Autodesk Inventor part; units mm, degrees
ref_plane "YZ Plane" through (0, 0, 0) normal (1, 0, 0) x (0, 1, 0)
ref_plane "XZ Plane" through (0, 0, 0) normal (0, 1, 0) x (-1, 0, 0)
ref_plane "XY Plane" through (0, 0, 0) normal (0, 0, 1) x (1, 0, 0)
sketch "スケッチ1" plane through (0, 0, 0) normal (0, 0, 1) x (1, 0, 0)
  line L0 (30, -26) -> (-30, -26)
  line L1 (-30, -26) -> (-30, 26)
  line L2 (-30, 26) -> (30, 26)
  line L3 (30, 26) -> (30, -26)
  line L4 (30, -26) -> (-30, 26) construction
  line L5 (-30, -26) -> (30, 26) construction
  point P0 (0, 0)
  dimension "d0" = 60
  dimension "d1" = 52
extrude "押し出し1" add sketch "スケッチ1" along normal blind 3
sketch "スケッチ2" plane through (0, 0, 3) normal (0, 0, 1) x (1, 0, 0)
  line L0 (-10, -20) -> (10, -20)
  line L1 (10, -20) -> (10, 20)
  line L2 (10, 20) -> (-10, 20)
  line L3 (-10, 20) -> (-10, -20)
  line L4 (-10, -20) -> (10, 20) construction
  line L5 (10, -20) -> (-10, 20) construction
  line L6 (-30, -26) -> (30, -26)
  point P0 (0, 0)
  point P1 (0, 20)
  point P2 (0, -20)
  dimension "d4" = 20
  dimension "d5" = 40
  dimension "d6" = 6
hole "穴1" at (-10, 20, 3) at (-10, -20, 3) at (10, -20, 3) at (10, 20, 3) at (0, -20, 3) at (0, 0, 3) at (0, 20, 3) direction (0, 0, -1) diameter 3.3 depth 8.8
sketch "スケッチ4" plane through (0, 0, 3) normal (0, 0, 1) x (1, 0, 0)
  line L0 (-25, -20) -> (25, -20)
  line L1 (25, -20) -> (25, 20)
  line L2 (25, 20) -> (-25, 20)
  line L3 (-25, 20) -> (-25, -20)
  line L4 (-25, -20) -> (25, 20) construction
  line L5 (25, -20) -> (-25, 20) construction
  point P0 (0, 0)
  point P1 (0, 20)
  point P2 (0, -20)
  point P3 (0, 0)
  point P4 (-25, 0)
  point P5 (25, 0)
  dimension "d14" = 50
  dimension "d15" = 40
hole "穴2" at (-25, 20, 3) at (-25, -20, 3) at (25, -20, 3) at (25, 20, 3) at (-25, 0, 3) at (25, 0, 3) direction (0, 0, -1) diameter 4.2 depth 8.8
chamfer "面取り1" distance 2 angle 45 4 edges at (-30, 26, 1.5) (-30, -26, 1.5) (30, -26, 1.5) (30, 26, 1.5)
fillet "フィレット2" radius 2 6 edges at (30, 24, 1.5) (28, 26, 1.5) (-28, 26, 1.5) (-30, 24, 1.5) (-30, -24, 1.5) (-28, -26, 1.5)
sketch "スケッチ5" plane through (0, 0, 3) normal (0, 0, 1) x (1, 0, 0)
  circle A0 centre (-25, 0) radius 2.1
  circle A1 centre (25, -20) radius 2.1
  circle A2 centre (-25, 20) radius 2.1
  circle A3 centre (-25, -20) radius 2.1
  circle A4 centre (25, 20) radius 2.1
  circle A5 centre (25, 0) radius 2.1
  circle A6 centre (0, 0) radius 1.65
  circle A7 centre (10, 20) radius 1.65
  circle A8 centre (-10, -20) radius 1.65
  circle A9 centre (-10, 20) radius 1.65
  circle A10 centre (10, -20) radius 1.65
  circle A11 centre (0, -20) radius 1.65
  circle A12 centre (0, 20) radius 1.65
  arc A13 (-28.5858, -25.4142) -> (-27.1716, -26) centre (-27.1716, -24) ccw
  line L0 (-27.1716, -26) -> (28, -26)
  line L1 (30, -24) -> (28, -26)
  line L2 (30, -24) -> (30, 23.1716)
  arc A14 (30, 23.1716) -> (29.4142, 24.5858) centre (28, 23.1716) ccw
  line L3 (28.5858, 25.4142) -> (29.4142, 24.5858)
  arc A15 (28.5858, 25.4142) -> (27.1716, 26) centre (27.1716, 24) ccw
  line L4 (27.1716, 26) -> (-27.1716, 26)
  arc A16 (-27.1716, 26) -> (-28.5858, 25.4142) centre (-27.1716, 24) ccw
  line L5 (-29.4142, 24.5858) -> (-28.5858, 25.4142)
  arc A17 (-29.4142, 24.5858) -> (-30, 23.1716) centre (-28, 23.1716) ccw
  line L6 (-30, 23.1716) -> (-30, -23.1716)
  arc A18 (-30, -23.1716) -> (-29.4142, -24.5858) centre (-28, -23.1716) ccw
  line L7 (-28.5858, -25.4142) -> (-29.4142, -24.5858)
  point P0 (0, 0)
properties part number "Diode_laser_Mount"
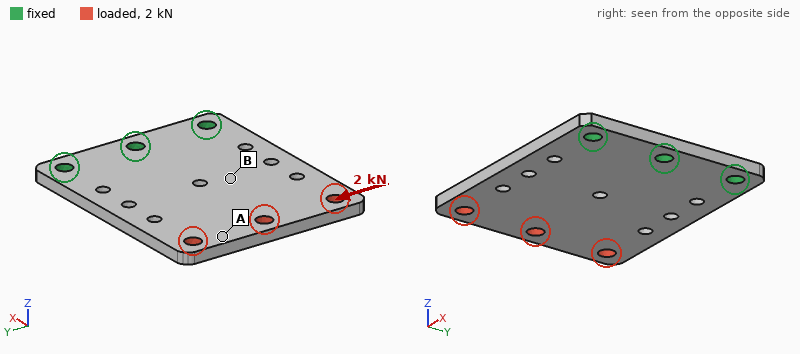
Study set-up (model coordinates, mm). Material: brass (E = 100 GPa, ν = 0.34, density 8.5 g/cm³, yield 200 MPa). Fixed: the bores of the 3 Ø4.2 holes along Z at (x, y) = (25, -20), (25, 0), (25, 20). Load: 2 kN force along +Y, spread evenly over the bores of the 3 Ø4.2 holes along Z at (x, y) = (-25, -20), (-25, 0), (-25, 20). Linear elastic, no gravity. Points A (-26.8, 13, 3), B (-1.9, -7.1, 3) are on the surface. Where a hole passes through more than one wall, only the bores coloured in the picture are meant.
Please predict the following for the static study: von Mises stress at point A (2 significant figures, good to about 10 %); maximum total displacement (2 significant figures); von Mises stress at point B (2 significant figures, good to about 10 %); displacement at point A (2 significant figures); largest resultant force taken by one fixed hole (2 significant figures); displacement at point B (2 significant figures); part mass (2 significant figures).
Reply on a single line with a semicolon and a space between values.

16 MPa; 59 µm; 35 MPa; 52 µm; 2.5 kN; 21 µm; 76 g
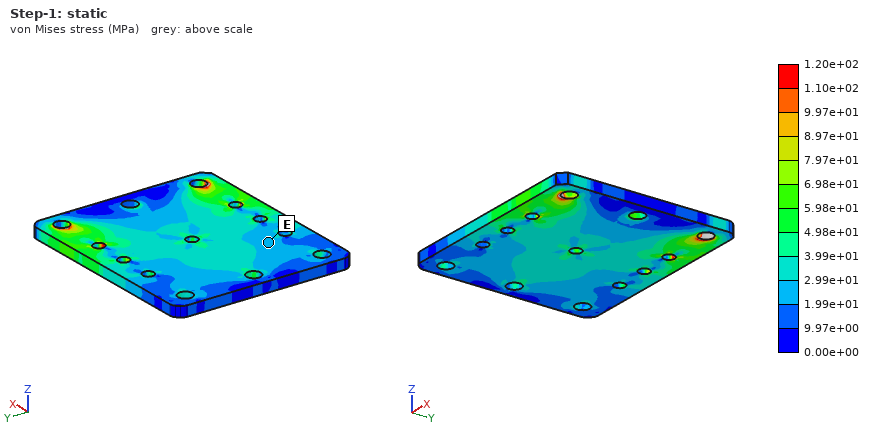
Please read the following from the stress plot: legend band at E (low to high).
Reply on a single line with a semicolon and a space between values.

1.99e+01 to 2.99e+01 MPa
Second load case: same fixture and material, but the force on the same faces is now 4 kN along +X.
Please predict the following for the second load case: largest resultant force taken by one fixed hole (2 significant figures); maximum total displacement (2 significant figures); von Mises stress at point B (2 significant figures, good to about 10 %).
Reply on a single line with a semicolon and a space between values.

1.4 kN; 19 µm; 26 MPa
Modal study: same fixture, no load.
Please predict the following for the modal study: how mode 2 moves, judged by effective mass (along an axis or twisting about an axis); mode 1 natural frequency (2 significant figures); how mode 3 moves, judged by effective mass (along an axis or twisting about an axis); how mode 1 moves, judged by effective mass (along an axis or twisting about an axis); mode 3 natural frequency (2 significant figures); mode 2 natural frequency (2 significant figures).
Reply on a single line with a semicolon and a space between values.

twisting about X; 580 Hz; along Z; along Z; 3500 Hz; 1400 Hz
